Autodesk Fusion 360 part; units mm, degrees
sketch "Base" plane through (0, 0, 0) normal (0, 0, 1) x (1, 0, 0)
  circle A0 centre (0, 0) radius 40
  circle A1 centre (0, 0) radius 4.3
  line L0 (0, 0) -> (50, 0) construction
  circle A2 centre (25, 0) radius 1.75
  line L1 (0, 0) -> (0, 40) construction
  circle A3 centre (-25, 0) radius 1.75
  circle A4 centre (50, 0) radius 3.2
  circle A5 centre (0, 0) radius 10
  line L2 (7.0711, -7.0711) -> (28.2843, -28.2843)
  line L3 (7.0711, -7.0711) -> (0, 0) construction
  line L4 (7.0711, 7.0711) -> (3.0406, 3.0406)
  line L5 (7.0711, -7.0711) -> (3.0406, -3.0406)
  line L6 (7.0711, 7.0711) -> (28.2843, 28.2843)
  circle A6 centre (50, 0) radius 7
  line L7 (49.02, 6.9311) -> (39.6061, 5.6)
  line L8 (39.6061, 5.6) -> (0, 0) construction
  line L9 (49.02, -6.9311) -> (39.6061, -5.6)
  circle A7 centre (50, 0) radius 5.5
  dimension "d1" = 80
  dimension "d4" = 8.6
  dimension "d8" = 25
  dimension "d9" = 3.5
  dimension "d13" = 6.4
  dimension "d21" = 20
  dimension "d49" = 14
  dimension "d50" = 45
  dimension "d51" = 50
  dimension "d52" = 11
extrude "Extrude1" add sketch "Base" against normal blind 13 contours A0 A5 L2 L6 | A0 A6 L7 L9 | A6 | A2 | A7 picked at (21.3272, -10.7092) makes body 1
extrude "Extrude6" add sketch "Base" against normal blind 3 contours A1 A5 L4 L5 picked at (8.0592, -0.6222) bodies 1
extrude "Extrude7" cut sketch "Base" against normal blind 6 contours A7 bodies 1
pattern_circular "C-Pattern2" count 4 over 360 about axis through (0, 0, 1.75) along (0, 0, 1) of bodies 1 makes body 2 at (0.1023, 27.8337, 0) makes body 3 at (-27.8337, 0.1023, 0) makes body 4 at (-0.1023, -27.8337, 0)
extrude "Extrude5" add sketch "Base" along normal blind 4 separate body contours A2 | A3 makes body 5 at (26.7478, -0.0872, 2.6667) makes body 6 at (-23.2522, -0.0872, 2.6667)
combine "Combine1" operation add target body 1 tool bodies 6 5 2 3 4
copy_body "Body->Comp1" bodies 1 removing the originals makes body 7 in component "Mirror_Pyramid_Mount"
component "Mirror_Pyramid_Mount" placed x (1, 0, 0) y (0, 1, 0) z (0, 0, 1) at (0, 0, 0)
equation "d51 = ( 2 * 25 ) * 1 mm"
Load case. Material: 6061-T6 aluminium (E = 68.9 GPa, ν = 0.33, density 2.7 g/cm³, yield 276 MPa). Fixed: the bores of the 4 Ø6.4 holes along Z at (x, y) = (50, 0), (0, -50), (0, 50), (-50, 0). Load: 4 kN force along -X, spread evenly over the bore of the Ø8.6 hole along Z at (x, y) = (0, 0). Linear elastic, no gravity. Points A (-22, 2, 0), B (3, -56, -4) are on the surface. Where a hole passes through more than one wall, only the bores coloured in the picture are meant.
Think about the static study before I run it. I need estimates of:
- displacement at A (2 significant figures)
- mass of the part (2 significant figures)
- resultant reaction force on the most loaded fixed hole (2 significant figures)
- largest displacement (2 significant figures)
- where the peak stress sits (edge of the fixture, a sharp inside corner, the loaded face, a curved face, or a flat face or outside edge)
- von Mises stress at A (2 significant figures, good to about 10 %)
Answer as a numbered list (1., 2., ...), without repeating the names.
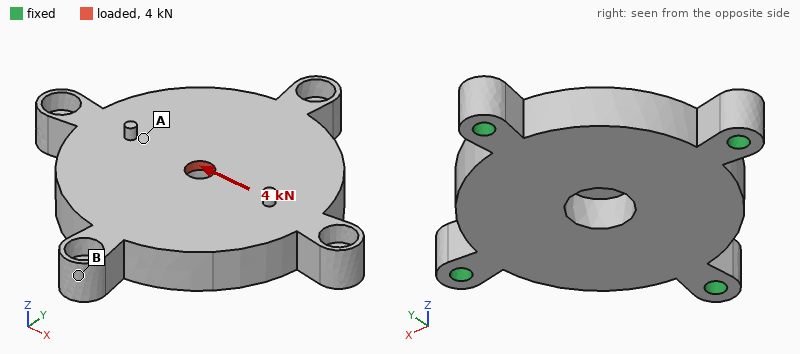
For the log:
1. 4.3 µm
2. 190 g
3. 1.6 kN
4. 11 µm
5. the loaded face
6. 12 MPa
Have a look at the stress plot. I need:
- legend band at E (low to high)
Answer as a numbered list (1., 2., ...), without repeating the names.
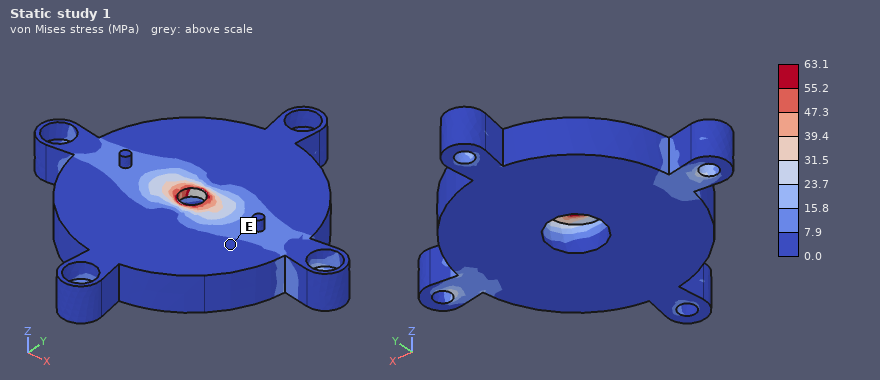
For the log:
1. 0.0 to 7.9 MPa
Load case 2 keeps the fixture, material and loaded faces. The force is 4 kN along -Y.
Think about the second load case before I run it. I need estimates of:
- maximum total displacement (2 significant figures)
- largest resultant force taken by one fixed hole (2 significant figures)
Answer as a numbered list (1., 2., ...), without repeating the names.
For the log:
1. 11 µm
2. 1.6 kN
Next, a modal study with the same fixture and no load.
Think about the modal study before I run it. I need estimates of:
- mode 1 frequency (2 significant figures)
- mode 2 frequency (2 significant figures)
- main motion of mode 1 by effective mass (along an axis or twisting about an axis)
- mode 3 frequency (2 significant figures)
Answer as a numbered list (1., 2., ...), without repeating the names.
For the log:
1. 6000 Hz
2. 9100 Hz
3. along Z
4. 9100 Hz
